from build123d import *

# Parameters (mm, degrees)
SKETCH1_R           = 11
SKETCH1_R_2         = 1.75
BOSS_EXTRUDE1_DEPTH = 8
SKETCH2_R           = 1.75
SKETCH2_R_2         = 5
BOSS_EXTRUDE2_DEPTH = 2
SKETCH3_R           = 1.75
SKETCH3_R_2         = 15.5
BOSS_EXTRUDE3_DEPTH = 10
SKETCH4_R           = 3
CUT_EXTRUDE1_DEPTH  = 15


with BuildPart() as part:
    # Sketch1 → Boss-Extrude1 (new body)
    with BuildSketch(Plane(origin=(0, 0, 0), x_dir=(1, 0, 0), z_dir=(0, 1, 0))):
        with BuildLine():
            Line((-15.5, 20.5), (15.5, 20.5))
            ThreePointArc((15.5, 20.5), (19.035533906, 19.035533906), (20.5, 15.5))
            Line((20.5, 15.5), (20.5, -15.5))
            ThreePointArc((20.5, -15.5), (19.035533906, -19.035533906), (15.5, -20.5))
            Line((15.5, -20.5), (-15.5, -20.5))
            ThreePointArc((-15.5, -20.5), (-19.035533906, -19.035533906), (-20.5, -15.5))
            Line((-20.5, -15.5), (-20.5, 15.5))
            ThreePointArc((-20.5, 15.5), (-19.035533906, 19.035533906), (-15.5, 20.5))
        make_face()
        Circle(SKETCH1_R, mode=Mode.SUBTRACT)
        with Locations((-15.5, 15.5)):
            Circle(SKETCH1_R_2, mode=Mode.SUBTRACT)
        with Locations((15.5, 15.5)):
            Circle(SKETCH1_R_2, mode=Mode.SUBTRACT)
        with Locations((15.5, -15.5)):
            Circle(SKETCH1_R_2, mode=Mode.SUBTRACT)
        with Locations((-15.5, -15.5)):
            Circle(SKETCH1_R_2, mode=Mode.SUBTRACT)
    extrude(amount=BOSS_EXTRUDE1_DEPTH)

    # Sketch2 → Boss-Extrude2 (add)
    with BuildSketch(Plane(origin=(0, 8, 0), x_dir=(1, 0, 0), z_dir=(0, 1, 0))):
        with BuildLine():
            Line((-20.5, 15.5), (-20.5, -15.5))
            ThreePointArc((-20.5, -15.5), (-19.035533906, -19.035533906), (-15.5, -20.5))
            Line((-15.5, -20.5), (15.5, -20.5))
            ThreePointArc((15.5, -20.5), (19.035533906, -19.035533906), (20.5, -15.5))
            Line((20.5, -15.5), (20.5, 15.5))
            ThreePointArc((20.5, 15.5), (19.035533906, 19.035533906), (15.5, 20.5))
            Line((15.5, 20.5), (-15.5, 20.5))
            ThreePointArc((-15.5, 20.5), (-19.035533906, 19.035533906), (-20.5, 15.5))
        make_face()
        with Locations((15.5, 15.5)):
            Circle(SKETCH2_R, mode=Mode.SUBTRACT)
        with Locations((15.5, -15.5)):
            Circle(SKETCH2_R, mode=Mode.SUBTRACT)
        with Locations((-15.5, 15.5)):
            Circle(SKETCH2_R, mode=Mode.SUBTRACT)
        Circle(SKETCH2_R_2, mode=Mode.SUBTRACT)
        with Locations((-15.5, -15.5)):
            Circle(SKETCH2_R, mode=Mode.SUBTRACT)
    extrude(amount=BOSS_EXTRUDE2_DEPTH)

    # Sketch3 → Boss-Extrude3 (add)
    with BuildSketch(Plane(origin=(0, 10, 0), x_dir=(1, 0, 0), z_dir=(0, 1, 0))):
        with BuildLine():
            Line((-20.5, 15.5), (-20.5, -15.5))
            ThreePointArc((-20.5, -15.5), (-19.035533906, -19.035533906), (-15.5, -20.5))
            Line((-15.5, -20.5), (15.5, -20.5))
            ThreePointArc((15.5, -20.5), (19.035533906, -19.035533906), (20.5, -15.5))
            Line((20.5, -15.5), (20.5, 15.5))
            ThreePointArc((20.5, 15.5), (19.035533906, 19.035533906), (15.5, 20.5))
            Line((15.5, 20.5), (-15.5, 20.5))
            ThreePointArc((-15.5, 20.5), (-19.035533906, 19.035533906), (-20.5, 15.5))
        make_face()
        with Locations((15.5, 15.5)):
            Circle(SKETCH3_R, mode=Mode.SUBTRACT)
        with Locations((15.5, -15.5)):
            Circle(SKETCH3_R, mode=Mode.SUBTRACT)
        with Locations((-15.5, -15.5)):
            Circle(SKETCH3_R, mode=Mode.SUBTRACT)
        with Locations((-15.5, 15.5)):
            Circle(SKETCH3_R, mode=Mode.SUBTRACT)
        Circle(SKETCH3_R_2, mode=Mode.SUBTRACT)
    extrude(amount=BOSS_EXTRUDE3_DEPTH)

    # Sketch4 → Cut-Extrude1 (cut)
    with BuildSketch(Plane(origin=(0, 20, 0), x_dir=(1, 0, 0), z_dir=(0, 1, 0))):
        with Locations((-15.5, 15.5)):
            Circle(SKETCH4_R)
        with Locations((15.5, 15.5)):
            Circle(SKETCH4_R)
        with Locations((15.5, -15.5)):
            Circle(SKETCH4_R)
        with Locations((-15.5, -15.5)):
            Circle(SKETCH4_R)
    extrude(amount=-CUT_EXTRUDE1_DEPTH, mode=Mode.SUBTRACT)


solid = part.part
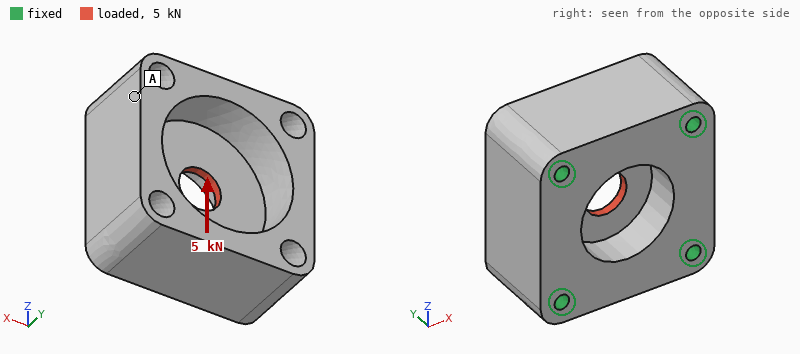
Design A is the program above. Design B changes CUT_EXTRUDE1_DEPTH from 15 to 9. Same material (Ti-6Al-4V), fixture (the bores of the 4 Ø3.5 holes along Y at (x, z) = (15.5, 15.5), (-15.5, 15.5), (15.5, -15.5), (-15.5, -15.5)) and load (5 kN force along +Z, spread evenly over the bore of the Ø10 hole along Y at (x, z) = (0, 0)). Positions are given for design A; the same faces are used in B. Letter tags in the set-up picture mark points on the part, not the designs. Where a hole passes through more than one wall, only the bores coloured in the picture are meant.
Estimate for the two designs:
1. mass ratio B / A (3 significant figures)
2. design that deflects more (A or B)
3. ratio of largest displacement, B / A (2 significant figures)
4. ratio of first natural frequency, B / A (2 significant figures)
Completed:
1.02
A
0.85
1.2
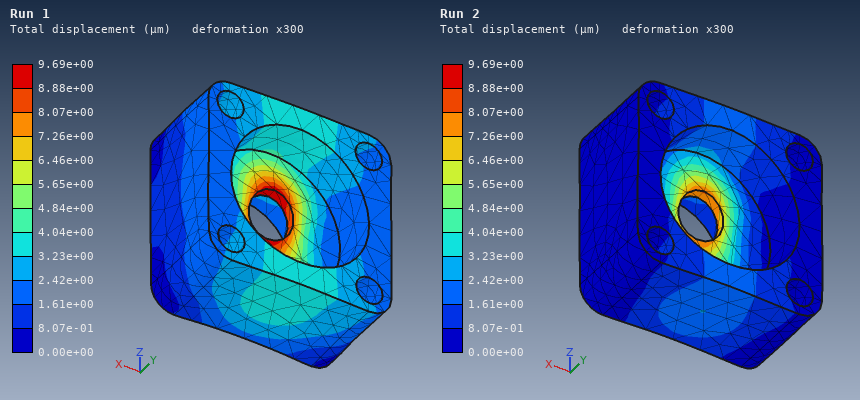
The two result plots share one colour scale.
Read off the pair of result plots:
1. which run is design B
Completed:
Run 2
